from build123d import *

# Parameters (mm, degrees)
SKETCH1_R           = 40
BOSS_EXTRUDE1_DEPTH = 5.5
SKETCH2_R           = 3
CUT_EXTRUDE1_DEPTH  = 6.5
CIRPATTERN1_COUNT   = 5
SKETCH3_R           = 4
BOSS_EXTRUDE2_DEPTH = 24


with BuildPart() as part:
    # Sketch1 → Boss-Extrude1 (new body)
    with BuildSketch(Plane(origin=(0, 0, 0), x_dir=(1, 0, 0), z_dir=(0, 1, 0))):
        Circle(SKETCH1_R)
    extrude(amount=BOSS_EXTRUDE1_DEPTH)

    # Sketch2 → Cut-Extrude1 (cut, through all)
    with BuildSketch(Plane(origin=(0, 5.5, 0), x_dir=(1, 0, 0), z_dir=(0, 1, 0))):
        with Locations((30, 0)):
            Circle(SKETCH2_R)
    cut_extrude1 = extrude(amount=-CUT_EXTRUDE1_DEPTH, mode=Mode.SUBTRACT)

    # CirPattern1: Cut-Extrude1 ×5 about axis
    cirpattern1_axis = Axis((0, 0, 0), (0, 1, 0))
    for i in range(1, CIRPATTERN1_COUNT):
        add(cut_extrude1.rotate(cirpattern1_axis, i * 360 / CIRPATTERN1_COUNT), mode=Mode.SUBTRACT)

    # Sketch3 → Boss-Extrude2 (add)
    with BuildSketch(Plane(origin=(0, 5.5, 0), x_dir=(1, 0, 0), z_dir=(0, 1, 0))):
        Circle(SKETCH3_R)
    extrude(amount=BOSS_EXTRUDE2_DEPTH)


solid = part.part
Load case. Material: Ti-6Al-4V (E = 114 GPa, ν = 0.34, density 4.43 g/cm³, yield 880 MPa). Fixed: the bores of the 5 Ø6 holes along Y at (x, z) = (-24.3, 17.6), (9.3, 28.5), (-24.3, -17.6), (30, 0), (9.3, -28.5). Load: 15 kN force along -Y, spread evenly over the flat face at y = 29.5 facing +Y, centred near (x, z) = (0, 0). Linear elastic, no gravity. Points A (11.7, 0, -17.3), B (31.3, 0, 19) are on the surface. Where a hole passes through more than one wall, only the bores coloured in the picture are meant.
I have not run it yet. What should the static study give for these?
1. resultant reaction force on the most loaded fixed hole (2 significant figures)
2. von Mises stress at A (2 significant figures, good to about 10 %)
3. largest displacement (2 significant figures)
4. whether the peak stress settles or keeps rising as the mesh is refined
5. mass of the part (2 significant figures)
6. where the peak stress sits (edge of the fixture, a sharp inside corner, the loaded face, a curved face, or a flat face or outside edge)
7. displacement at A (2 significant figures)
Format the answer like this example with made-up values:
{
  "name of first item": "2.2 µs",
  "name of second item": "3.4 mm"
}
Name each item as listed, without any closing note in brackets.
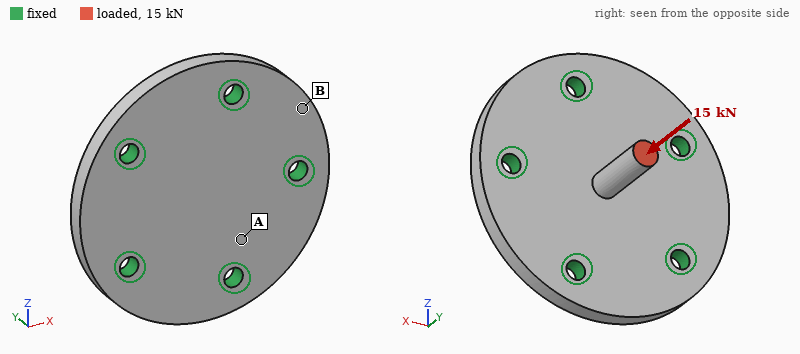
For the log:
{
  "resultant reaction force on the most loaded fixed hole": "3.0 kN",
  "von Mises stress at A": "130 MPa",
  "largest displacement": "0.23 mm",
  "whether the peak stress settles or keeps rising as the mesh is refined": "keeps rising",
  "mass of the part": "120 g",
  "where the peak stress sits": "edge of the fixture",
  "displacement at A": "0.039 mm"
}
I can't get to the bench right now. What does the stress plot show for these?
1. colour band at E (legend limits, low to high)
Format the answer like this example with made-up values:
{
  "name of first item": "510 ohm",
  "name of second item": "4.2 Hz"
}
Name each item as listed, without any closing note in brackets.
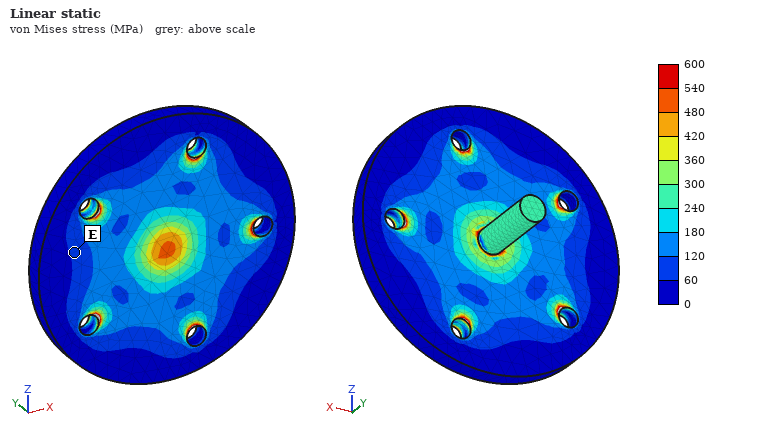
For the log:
{
  "colour band at E": "60 to 120 MPa"
}
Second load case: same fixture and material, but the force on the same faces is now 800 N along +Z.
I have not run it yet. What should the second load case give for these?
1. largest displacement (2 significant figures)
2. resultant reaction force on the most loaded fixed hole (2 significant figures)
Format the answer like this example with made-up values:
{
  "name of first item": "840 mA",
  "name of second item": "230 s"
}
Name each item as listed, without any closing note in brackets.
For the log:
{
  "largest displacement": "0.25 mm",
  "resultant reaction force on the most loaded fixed hole": "430 N"
}
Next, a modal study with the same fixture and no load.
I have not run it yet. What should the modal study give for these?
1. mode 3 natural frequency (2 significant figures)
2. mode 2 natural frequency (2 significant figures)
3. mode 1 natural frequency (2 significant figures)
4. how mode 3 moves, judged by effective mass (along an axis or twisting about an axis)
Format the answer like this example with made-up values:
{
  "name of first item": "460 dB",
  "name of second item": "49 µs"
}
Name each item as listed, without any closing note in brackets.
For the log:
{
  "mode 3 natural frequency": "11 kHz",
  "mode 2 natural frequency": "7400 Hz",
  "mode 1 natural frequency": "7400 Hz",
  "how mode 3 moves, judged by effective mass": "along Y"
}
